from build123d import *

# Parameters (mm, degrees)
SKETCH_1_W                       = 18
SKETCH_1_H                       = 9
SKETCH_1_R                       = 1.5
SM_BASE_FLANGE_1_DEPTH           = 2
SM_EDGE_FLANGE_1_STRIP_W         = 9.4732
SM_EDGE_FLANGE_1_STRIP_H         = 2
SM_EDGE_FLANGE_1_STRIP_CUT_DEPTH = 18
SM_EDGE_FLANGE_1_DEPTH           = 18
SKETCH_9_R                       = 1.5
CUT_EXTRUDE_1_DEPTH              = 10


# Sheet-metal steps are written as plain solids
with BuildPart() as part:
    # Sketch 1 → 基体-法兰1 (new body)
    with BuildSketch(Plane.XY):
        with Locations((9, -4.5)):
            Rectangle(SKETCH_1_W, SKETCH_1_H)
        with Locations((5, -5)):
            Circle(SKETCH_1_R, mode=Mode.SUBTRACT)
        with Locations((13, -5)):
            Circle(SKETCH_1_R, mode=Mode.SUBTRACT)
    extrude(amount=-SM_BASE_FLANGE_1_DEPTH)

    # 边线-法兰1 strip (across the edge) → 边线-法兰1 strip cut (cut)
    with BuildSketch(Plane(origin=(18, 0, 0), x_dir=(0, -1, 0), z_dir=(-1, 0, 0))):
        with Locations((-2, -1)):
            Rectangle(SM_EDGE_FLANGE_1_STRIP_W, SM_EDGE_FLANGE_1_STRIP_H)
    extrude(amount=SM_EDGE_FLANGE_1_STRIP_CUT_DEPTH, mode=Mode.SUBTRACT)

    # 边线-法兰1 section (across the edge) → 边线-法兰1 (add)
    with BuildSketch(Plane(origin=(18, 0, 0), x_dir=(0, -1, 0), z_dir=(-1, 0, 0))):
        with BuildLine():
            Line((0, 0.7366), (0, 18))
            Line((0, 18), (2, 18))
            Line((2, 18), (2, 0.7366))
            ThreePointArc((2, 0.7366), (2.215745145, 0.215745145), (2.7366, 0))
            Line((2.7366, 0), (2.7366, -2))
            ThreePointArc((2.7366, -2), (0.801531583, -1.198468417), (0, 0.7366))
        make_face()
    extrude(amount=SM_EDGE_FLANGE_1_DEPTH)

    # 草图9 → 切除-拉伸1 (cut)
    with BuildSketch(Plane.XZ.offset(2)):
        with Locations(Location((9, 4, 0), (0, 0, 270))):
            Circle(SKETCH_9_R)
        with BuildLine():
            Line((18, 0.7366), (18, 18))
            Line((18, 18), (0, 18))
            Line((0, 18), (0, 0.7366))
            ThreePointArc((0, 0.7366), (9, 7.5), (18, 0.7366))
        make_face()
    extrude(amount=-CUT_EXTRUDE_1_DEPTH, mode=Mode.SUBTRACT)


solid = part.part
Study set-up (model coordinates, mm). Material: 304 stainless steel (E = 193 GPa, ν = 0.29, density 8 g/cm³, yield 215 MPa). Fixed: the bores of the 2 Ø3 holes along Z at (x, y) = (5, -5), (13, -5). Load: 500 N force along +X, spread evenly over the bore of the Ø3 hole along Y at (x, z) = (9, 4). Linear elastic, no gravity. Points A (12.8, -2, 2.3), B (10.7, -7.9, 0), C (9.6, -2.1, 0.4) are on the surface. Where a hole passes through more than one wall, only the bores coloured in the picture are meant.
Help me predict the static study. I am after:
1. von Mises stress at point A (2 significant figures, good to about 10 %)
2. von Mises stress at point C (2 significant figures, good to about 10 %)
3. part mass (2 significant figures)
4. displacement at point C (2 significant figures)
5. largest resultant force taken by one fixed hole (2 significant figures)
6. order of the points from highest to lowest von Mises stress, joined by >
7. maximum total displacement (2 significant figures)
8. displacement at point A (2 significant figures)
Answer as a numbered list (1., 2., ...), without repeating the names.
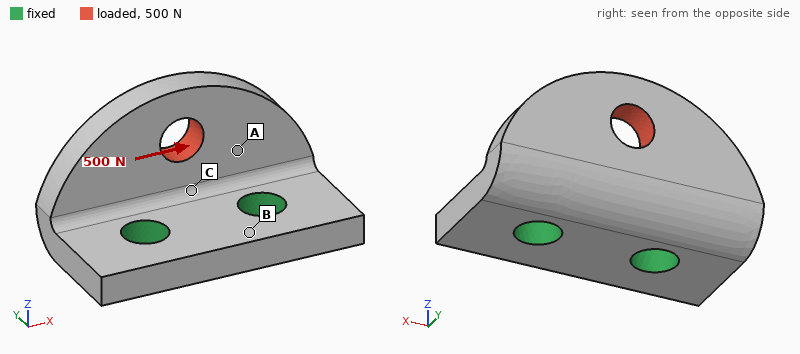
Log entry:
1. 49 MPa
2. 130 MPa
3. 3.7 g
4. 1.3 µm
5. 380 N
6. C > A > B
7. 6.9 µm
8. 3.6 µm
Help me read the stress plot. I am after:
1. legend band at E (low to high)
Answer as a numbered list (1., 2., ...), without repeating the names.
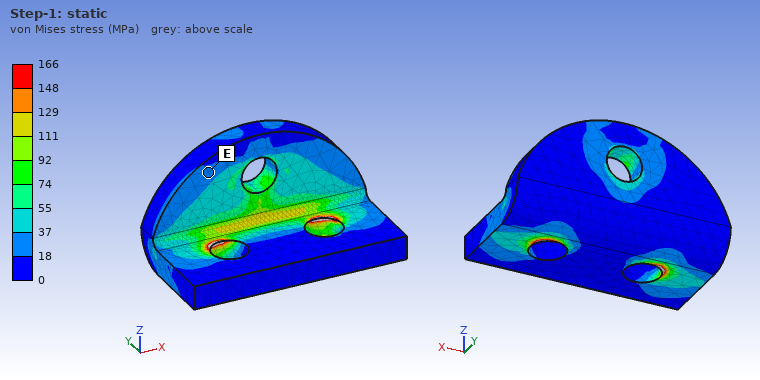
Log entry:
1. 18 to 37 MPa
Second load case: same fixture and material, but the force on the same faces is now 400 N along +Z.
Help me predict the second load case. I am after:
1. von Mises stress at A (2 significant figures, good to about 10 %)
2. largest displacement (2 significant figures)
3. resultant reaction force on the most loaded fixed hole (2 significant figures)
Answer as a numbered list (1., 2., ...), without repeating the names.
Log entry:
1. 18 MPa
2. 10 µm
3. 200 N
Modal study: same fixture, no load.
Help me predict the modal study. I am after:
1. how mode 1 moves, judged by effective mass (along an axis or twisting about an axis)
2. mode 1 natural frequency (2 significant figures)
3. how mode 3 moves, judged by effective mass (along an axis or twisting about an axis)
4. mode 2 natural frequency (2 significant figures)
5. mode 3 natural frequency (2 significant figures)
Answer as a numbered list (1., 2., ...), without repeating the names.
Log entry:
1. along Y
2. 19 kHz
3. along X
4. 32 kHz
5. 50 kHz
